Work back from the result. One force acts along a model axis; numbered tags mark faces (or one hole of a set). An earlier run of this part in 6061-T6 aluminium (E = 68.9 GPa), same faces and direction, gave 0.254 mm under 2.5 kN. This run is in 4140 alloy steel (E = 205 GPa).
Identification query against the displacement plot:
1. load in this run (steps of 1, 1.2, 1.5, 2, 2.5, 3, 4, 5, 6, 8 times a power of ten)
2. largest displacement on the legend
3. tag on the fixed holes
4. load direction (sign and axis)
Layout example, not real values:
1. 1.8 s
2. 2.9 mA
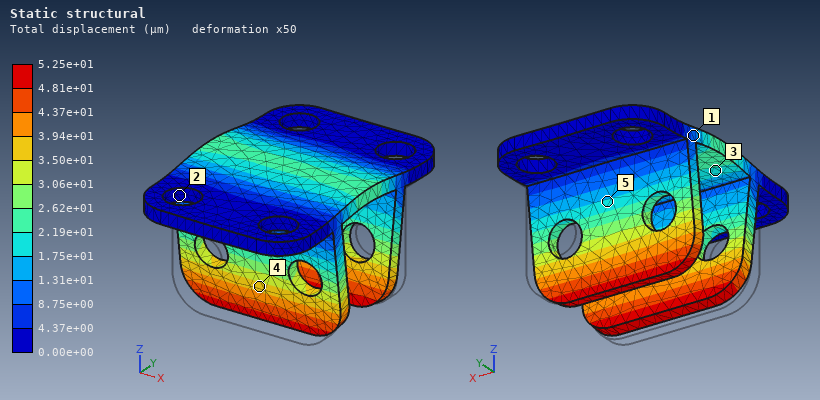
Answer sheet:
1. 1.5 kN
2. 5.25e+01 µm
3. 2
4. +Z
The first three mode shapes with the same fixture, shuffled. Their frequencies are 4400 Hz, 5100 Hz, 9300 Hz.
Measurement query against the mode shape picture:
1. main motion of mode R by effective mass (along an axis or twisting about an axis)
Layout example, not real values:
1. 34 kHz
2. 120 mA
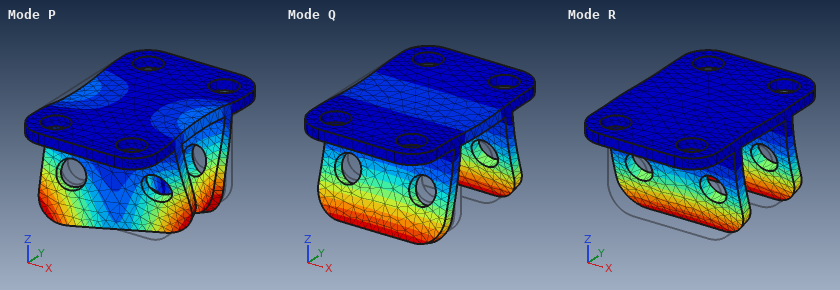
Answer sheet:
1. along Y
